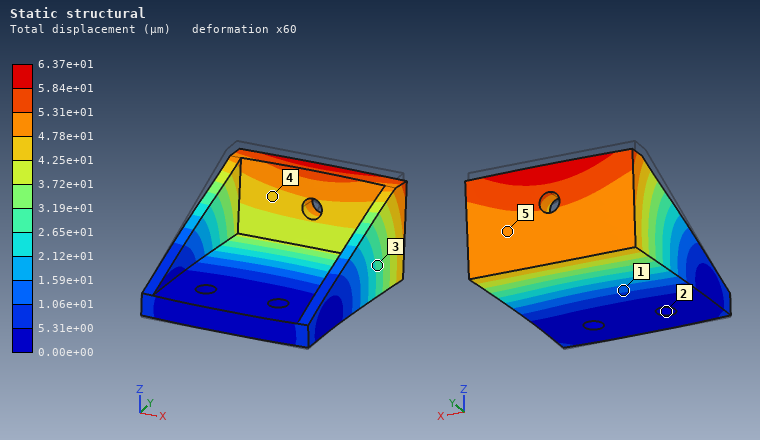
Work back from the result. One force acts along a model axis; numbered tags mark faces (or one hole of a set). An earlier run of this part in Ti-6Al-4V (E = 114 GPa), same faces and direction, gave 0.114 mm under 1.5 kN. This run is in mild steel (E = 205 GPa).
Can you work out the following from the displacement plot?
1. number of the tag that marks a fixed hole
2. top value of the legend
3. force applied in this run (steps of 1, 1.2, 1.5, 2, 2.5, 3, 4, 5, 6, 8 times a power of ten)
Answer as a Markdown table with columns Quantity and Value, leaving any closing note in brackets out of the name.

| Quantity | Value |
|---|---|
| number of the tag that marks a fixed hole | 2 |
| top value of the legend | 6.37e+01 µm |
| force applied in this run | 1.5 kN |
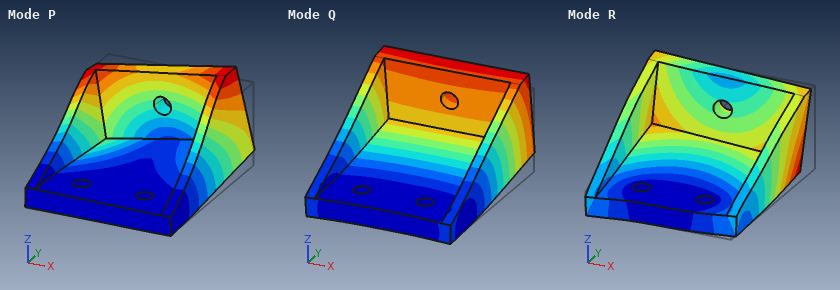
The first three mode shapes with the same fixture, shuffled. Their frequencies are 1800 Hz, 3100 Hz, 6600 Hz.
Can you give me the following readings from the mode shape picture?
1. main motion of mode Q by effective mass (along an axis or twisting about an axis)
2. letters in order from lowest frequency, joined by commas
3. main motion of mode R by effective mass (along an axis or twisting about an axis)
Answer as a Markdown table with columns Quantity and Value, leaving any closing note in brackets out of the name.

| Quantity | Value |
|---|---|
| main motion of mode Q by effective mass | along Z |
| letters in order from lowest frequency, joined by commas | Q, P, R |
| main motion of mode R by effective mass | along X |
